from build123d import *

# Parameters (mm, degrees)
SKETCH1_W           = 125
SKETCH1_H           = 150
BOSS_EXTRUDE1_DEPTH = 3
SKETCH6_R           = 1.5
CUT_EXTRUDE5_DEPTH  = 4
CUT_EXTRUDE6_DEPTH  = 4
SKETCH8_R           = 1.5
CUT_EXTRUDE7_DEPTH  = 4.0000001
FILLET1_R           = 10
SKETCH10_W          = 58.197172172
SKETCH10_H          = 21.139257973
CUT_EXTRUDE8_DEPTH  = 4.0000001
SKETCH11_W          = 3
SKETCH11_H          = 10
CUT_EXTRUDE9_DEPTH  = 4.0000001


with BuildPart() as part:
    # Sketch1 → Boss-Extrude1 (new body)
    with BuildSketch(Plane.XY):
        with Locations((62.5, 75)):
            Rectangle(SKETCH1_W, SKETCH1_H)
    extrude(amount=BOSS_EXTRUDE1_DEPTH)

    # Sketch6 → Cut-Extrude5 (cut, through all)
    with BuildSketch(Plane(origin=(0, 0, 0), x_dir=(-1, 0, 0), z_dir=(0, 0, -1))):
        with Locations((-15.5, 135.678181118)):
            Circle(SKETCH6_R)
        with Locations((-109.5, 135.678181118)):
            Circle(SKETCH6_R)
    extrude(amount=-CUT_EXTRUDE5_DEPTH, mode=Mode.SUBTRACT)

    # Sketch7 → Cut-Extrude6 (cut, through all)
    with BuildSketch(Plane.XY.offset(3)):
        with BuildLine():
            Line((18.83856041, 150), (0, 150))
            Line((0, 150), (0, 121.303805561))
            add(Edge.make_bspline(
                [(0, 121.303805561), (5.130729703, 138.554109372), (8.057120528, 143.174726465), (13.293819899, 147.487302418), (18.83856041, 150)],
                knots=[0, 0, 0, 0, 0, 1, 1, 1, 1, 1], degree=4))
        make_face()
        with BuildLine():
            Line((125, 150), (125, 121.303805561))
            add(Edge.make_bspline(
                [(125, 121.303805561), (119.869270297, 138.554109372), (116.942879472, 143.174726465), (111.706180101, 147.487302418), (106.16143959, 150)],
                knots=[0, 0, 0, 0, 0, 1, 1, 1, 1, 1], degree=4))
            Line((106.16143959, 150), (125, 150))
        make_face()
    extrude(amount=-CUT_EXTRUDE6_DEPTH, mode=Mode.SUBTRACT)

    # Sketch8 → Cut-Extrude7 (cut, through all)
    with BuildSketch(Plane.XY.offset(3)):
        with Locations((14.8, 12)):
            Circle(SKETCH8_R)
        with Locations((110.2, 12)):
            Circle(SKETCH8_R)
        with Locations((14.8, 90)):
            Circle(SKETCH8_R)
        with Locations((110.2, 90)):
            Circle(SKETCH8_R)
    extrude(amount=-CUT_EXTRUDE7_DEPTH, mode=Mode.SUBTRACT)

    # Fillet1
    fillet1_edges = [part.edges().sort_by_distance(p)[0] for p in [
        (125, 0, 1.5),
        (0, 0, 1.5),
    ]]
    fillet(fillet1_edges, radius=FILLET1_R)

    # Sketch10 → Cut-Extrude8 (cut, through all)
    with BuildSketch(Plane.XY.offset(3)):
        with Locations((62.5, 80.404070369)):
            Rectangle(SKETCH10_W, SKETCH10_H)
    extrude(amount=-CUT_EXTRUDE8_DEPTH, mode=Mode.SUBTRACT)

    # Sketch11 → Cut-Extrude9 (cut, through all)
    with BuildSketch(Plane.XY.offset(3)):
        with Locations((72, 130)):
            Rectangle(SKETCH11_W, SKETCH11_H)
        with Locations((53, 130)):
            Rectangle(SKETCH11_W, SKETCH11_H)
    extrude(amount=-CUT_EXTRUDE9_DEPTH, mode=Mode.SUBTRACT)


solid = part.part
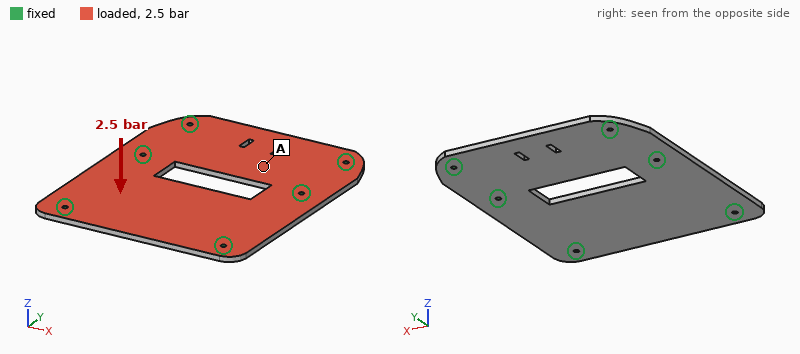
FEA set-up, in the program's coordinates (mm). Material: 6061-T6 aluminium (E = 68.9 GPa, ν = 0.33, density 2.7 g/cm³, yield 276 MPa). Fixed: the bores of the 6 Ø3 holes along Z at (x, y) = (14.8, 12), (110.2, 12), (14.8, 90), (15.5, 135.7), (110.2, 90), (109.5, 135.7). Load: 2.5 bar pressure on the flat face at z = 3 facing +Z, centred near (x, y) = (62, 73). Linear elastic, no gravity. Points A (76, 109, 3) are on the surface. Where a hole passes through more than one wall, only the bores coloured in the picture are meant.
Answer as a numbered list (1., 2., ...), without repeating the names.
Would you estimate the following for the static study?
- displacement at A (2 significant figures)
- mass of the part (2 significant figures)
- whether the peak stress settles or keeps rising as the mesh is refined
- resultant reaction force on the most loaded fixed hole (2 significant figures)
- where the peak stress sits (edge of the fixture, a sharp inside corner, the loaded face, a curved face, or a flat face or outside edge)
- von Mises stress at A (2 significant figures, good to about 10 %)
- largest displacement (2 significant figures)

1. 0.36 mm
2. 140 g
3. keeps rising
4. 880 N
5. edge of the fixture
6. 50 MPa
7. 0.72 mm
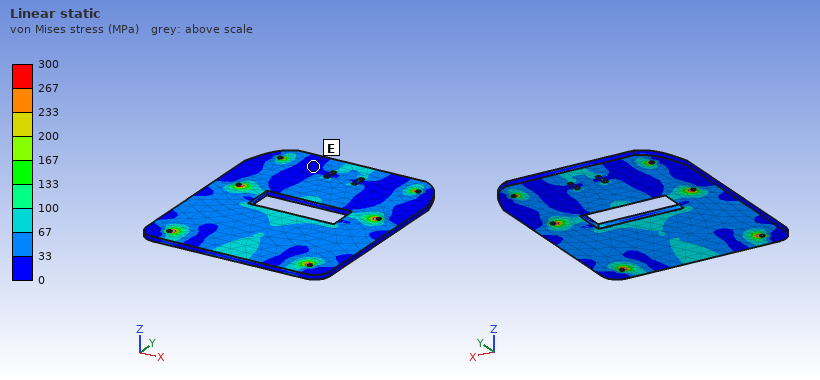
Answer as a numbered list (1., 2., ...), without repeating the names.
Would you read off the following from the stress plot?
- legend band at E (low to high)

1. 0 to 33 MPa
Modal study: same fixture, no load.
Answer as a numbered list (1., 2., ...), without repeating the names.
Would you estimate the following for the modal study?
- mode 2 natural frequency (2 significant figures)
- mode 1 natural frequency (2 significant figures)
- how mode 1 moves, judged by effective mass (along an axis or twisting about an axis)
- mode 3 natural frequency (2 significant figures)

1. 1600 Hz
2. 1300 Hz
3. along Z
4. 2100 Hz
